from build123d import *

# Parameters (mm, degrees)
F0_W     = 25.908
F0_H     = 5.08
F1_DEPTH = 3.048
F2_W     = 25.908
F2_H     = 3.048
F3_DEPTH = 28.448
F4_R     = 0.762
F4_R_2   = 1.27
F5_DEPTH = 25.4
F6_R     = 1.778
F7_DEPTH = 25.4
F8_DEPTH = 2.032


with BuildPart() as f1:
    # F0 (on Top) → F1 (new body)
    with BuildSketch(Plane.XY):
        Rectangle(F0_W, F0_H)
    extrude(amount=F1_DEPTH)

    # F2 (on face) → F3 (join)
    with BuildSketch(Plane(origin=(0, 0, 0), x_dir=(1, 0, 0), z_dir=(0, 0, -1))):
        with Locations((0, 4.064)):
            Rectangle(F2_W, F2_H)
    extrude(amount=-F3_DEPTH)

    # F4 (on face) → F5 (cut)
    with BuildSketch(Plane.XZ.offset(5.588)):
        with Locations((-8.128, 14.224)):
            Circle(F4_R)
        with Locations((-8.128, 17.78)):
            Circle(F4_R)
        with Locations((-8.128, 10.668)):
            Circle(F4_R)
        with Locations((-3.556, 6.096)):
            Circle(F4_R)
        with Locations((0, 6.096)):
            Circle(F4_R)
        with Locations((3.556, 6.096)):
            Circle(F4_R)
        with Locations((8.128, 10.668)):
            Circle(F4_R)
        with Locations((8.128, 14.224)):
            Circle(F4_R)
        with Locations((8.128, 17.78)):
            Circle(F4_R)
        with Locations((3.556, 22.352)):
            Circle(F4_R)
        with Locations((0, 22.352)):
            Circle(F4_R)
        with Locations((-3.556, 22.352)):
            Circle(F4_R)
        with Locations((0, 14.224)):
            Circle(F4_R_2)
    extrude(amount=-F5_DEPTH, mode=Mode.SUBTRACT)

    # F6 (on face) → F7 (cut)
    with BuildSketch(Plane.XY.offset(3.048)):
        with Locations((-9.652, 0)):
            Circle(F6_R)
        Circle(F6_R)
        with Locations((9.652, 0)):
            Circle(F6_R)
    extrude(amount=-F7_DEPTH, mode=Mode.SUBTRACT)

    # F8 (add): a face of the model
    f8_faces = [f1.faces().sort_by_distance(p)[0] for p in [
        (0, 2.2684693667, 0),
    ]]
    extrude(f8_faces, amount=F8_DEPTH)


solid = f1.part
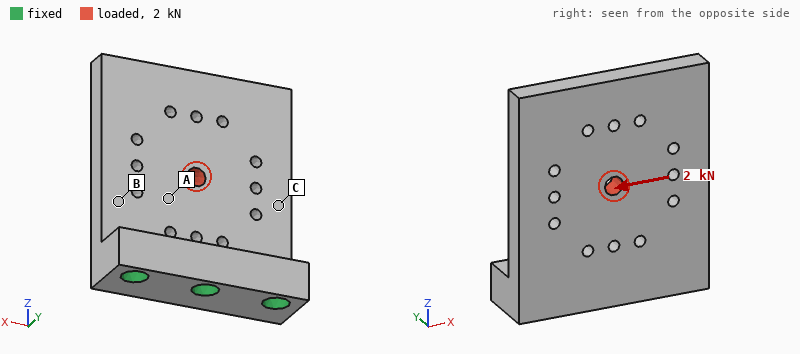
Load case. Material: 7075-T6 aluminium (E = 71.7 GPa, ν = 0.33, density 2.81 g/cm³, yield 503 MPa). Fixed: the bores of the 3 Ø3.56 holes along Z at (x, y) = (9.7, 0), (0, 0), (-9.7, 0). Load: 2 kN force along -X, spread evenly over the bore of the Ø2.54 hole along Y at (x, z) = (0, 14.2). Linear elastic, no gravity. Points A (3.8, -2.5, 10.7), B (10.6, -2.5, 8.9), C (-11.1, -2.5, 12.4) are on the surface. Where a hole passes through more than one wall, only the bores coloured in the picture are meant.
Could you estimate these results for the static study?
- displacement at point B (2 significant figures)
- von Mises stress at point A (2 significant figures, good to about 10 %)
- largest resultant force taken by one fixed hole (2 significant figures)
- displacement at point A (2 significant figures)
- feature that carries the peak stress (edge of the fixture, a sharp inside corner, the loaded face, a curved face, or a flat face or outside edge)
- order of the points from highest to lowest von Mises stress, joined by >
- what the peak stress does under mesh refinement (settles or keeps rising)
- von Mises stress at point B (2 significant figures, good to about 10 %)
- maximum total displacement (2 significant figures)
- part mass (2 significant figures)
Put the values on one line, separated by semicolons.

20 µm; 72 MPa; 1.4 kN; 21 µm; edge of the fixture; A > B > C; keeps rising; 47 MPa; 47 µm; 8.0 g
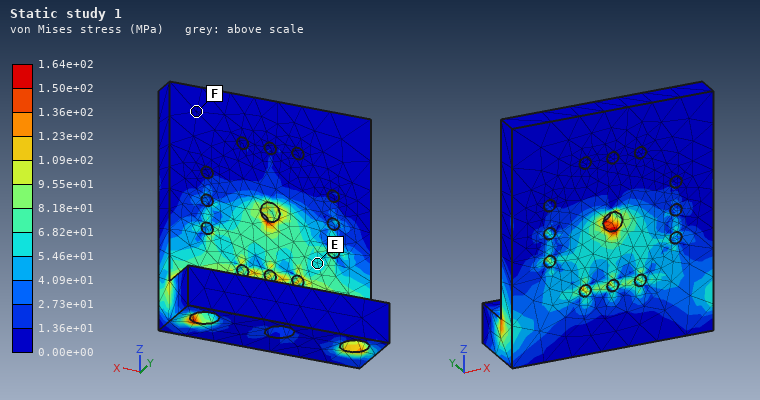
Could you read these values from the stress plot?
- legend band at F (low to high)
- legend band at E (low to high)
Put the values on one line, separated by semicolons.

0.00e+00 to 1.36e+01 MPa; 5.46e+01 to 6.82e+01 MPa
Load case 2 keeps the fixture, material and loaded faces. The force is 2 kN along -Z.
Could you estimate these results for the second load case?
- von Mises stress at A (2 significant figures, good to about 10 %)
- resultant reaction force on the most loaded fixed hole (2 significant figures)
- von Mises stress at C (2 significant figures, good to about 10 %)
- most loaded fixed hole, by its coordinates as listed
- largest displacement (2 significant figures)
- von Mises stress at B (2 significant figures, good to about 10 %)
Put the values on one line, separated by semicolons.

37 MPa; 750 N; 13 MPa; (0, 0); 29 µm; 17 MPa
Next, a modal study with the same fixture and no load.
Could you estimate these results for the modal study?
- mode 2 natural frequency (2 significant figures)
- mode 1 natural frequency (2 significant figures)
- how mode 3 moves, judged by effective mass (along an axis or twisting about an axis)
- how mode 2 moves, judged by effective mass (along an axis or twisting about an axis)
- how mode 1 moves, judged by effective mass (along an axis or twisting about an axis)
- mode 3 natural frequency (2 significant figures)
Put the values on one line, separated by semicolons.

7900 Hz; 3300 Hz; along X; twisting about Z; along Y; 15 kHz
